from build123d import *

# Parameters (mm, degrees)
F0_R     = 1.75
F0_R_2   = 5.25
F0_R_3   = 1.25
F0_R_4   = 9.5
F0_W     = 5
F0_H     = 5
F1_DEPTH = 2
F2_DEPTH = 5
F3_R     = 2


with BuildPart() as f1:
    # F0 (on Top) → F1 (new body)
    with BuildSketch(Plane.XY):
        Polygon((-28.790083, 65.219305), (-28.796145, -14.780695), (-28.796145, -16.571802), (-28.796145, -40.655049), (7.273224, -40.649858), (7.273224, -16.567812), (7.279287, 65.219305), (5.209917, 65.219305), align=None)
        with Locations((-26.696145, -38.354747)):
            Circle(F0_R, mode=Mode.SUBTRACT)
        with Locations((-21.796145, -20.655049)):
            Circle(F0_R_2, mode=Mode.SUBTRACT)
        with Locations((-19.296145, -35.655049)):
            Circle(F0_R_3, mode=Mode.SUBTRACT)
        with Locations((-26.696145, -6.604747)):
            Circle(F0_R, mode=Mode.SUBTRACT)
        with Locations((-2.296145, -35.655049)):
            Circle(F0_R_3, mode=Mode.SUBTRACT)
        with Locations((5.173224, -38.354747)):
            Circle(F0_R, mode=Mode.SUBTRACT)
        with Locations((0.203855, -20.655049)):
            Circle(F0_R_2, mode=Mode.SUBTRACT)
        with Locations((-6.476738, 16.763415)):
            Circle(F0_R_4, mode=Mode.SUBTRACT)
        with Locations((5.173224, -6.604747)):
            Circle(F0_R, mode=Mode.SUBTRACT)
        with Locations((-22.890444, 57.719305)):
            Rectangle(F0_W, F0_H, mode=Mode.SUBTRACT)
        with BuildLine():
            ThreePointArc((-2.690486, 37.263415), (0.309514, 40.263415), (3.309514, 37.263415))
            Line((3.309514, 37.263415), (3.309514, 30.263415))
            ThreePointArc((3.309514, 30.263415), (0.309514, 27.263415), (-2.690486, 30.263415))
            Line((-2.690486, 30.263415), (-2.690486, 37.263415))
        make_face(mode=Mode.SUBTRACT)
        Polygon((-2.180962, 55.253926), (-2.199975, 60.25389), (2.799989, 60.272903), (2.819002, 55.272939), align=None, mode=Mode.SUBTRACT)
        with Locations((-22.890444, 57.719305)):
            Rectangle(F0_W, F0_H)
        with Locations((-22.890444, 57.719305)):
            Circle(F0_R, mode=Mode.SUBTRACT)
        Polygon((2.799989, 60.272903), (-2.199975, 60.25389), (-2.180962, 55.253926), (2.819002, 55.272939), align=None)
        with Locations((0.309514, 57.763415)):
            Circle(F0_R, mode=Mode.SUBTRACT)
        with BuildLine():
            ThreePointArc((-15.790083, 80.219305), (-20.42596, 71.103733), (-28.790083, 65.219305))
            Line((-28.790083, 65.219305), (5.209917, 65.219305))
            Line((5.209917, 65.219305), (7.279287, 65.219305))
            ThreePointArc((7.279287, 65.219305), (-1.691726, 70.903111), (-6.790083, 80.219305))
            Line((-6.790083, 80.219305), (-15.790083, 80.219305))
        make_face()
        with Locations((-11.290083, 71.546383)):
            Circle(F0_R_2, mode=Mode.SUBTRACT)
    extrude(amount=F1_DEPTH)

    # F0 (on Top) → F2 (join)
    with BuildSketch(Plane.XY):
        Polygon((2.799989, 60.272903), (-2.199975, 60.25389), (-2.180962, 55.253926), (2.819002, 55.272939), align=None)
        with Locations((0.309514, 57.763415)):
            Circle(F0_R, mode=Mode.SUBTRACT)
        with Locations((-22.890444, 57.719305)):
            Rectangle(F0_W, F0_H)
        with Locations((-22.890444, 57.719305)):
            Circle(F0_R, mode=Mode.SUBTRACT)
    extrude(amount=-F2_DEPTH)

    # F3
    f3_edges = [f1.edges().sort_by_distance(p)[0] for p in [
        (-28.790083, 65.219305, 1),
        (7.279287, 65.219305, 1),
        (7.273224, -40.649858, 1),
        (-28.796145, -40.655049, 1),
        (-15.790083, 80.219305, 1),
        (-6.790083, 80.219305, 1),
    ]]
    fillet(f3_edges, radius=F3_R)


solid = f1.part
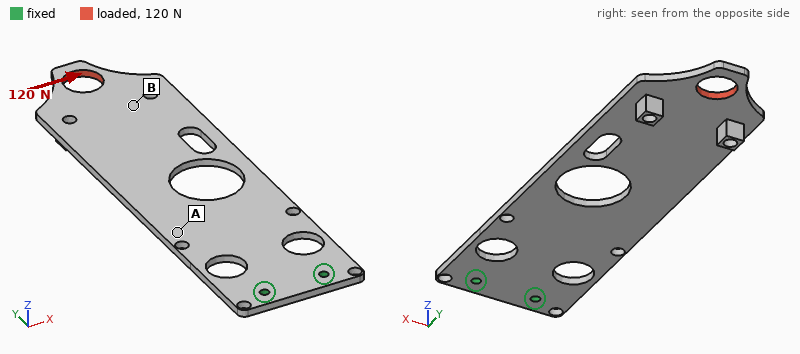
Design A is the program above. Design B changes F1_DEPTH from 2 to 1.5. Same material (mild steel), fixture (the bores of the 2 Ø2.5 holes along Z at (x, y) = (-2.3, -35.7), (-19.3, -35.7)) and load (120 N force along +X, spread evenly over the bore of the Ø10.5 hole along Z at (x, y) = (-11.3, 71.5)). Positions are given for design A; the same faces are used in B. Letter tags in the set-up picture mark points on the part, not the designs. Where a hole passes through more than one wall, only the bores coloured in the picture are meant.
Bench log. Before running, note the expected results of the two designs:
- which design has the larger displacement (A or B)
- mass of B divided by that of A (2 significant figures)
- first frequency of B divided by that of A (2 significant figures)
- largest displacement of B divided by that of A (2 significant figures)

B
0.76
0.75
1.3
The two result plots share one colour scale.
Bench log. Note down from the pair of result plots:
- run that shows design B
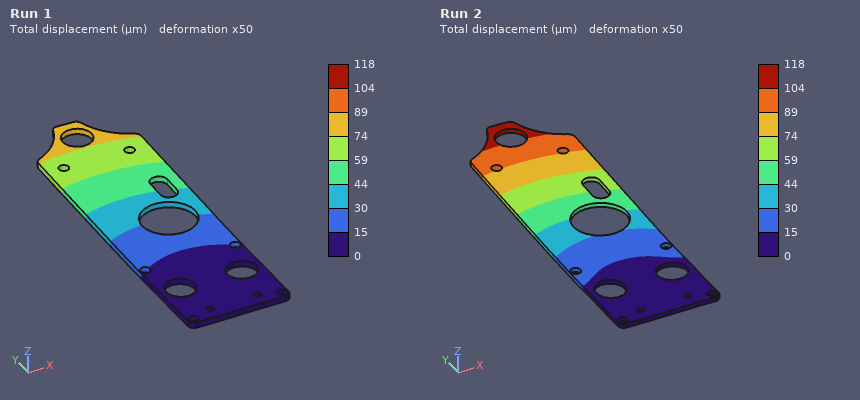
Run 2
